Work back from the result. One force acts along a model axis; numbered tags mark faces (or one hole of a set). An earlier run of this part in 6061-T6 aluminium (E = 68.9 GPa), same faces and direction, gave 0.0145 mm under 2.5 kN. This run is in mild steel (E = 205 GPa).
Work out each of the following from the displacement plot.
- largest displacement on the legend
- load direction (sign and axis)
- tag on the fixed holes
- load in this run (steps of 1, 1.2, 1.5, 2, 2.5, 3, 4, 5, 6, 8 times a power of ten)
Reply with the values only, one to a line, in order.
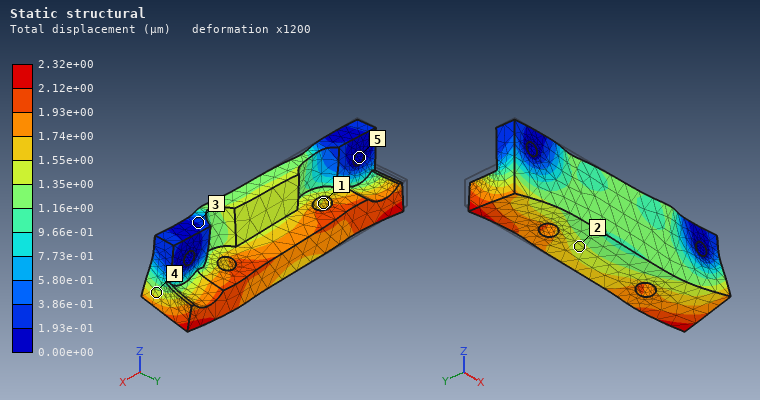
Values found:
2.32e+00 µm
+X
5
1.2 kN
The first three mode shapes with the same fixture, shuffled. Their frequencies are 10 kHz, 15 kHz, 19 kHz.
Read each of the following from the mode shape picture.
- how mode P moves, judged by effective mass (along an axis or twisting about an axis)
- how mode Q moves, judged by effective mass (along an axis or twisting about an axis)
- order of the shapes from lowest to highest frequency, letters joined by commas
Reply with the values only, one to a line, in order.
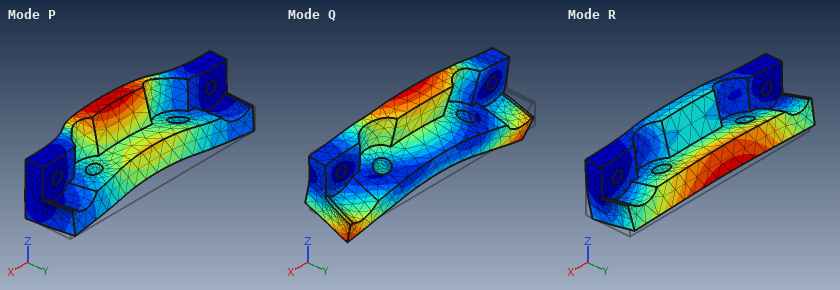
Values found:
along Y
along Z
R, P, Q
